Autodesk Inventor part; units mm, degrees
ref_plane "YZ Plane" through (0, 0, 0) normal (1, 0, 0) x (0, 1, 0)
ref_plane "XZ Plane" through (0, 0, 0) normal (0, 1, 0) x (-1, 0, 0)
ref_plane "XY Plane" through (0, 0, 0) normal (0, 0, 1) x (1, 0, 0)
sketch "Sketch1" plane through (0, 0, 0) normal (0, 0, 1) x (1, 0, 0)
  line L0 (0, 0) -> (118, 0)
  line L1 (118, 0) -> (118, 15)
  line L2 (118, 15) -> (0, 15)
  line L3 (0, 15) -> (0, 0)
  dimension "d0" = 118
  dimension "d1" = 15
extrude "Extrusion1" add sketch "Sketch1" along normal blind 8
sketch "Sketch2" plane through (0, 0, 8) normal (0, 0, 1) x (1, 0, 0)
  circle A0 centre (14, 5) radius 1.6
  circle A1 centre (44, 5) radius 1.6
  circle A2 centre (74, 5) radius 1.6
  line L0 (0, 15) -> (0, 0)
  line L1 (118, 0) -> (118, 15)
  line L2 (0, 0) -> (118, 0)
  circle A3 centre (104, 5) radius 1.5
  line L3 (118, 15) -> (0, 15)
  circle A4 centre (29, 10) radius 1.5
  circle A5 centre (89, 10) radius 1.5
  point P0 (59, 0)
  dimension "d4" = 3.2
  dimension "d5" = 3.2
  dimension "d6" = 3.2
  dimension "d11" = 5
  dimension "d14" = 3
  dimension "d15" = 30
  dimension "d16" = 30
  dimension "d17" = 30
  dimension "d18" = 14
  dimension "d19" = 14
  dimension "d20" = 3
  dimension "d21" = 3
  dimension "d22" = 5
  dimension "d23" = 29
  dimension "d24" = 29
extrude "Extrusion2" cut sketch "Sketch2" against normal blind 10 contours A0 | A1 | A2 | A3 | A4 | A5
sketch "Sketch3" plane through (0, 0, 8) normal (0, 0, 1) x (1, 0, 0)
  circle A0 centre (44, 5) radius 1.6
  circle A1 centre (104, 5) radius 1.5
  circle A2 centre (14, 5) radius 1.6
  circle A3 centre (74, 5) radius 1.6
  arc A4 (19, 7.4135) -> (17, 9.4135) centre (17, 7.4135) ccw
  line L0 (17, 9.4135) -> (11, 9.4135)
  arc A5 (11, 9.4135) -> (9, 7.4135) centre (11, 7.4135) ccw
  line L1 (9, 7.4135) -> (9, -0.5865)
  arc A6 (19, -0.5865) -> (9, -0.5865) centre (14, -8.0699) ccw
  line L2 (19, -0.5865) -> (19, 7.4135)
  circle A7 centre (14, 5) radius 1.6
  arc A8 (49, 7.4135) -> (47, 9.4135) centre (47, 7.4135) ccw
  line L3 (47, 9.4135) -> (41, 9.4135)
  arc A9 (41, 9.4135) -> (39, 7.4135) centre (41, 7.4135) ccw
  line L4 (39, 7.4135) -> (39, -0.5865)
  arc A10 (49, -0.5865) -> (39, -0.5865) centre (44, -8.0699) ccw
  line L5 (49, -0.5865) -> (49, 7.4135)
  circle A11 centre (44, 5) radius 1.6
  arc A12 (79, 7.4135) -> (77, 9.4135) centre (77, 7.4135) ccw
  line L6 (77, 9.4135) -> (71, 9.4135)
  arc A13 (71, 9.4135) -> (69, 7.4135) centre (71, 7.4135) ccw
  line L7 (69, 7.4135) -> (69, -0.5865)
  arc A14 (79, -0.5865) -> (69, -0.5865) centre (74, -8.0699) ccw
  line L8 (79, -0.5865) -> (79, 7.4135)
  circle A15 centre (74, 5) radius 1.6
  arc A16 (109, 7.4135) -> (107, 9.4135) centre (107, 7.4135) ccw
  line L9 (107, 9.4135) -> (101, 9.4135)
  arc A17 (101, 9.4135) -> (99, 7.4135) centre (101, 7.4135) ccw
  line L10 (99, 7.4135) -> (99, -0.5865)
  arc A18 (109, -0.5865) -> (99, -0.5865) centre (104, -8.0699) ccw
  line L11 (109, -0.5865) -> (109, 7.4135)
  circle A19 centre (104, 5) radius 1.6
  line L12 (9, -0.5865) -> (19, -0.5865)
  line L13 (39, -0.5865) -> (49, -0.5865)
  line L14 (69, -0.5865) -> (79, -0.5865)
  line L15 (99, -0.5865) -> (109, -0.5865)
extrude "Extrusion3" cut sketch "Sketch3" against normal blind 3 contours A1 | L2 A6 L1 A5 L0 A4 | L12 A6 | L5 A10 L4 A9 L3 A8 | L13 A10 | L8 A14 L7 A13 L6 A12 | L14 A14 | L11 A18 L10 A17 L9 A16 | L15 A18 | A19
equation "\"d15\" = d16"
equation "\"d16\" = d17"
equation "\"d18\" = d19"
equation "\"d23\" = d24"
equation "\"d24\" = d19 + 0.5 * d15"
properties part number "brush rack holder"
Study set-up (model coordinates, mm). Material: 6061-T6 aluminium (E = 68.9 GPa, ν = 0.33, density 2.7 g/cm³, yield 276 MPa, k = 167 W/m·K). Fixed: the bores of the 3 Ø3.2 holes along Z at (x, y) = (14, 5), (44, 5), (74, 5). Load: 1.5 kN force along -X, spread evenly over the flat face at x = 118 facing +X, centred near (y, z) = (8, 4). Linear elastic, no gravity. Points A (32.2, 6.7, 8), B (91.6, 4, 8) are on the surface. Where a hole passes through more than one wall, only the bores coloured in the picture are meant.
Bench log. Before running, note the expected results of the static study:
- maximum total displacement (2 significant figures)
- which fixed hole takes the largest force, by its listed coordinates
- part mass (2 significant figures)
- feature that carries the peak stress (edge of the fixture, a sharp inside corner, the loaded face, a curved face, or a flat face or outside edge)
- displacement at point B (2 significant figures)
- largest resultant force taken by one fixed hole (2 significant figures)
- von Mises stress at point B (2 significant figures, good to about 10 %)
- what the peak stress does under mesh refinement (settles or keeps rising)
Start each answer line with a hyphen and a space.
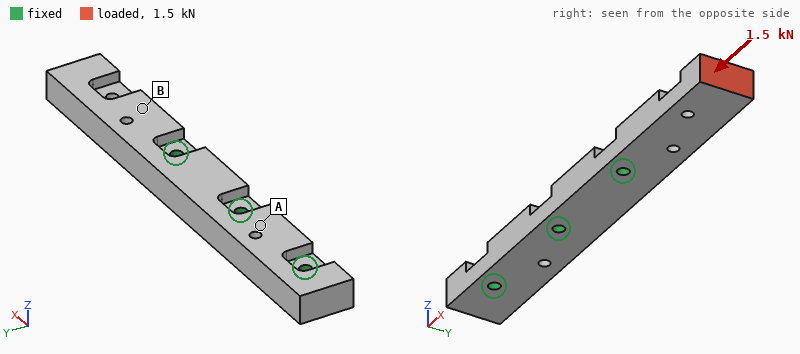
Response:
- 44 µm
- (74, 5)
- 35 g
- edge of the fixture
- 13 µm
- 1.2 kN
- 11 MPa
- keeps rising
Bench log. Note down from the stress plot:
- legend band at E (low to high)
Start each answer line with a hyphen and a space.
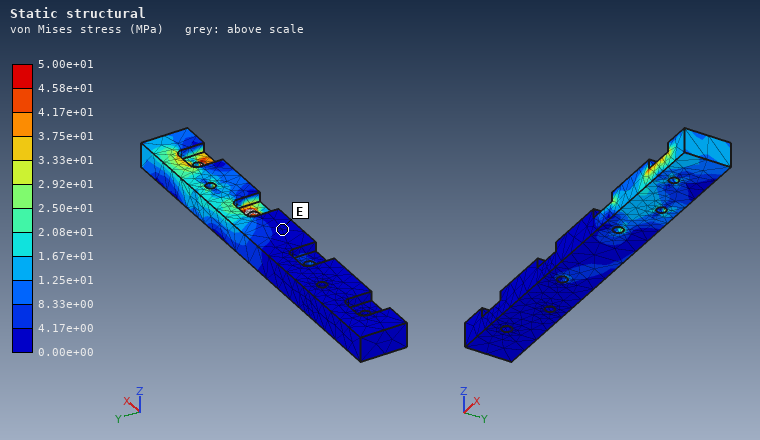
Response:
- 0.00e+00 to 4.17e+00 MPa
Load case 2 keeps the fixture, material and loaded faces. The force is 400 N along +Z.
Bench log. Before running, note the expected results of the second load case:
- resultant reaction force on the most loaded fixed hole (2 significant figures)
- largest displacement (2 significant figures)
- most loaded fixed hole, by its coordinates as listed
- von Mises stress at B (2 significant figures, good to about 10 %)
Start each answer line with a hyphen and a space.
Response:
- 750 N
- 0.49 mm
- (74, 5)
- 65 MPa
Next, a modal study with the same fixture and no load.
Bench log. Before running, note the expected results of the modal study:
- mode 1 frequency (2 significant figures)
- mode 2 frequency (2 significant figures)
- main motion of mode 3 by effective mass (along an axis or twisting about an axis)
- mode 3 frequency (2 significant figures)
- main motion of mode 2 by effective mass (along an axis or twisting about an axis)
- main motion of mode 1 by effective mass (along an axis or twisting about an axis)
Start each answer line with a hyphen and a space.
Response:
- 2500 Hz
- 4400 Hz
- twisting about X
- 11 kHz
- along Y
- along Z
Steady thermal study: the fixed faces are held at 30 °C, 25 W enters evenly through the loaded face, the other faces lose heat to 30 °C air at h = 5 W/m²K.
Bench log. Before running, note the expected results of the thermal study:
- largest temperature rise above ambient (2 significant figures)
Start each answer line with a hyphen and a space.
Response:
- 68 K
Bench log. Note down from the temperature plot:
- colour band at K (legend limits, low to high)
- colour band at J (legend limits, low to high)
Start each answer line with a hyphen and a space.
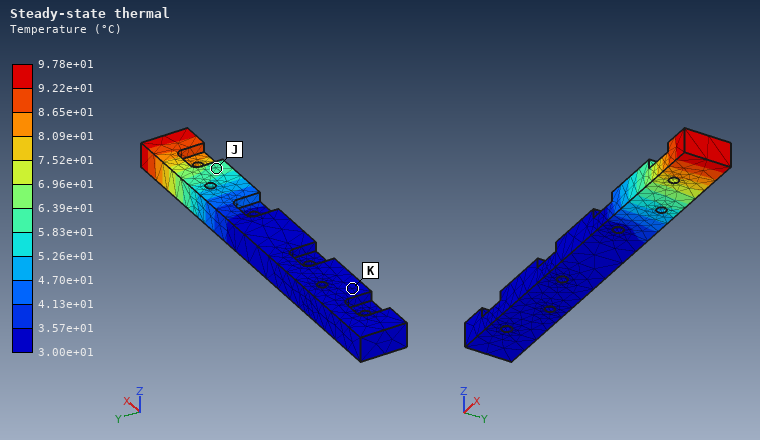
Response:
- 3.00e+01 to 3.57e+01 °C
- 5.83e+01 to 6.39e+01 °C
